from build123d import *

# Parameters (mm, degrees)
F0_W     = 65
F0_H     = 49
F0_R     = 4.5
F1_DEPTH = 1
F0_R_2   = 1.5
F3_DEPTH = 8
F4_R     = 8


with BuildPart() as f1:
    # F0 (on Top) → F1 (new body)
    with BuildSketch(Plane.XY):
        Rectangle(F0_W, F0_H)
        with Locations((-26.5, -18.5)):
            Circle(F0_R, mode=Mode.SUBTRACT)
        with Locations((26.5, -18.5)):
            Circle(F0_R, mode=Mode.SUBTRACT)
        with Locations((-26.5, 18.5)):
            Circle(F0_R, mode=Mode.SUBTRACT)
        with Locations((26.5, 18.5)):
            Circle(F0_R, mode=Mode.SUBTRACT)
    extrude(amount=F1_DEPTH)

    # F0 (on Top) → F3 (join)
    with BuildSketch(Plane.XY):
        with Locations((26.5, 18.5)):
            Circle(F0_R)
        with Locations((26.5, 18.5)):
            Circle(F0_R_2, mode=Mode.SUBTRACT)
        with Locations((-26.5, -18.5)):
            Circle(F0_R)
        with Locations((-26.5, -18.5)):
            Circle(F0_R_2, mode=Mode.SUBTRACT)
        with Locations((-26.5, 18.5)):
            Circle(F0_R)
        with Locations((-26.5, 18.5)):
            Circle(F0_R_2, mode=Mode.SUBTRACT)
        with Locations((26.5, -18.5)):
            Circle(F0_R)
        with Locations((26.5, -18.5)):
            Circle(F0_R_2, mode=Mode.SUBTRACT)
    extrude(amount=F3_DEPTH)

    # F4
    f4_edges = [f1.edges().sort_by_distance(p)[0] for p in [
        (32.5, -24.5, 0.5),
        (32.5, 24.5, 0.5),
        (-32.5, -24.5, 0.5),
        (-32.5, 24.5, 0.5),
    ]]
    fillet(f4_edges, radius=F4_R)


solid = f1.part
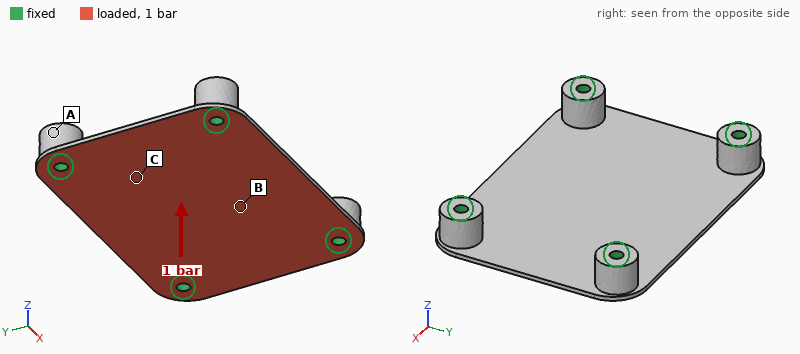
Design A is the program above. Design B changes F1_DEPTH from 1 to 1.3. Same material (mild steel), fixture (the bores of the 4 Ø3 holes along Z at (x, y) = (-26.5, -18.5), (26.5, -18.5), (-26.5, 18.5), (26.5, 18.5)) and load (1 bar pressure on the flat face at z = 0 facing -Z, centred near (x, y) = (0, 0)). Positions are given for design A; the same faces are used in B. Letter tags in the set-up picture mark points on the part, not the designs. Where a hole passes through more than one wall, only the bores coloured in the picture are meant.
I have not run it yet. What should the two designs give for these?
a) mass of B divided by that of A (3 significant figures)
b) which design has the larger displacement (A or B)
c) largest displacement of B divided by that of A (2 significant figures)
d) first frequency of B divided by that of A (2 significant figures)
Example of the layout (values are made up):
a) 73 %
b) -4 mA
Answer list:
a) 1.18
b) A
c) 0.47
d) 1.3
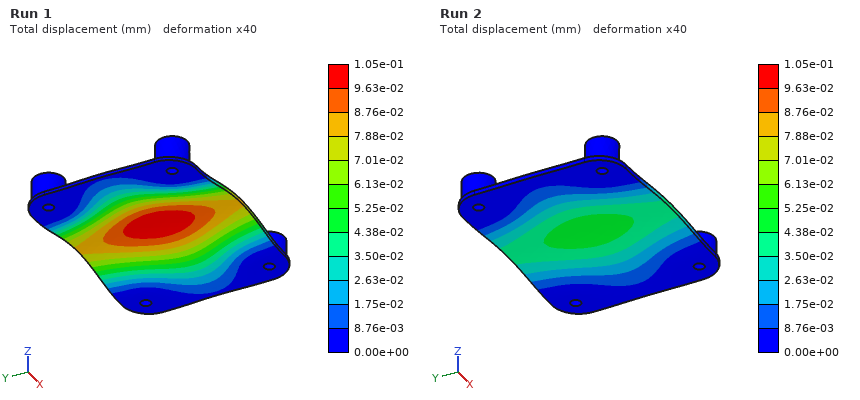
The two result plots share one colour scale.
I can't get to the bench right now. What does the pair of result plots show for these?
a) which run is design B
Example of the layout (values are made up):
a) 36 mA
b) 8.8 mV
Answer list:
a) Run 2
